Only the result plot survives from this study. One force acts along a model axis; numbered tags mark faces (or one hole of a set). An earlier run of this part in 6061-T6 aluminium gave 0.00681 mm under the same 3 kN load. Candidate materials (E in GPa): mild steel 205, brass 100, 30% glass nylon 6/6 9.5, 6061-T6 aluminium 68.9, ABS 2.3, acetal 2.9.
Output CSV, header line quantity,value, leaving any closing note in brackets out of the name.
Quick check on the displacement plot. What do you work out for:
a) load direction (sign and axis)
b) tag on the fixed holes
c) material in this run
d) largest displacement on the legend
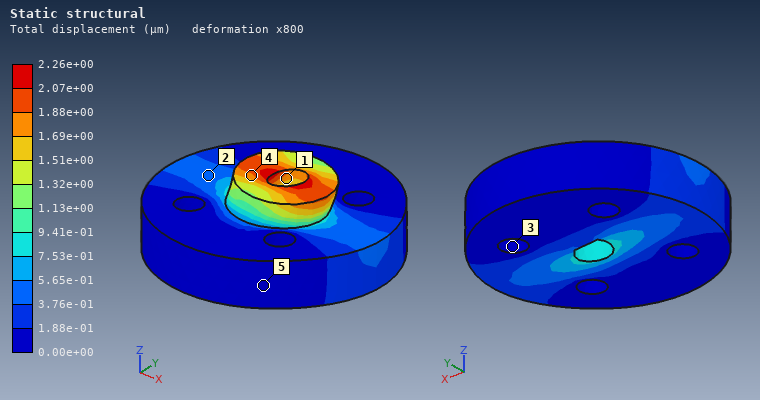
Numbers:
quantity,value
load direction,+X
tag on the fixed holes,3
material in this run,mild steel
largest displacement on the legend,2.26e+00 µm
